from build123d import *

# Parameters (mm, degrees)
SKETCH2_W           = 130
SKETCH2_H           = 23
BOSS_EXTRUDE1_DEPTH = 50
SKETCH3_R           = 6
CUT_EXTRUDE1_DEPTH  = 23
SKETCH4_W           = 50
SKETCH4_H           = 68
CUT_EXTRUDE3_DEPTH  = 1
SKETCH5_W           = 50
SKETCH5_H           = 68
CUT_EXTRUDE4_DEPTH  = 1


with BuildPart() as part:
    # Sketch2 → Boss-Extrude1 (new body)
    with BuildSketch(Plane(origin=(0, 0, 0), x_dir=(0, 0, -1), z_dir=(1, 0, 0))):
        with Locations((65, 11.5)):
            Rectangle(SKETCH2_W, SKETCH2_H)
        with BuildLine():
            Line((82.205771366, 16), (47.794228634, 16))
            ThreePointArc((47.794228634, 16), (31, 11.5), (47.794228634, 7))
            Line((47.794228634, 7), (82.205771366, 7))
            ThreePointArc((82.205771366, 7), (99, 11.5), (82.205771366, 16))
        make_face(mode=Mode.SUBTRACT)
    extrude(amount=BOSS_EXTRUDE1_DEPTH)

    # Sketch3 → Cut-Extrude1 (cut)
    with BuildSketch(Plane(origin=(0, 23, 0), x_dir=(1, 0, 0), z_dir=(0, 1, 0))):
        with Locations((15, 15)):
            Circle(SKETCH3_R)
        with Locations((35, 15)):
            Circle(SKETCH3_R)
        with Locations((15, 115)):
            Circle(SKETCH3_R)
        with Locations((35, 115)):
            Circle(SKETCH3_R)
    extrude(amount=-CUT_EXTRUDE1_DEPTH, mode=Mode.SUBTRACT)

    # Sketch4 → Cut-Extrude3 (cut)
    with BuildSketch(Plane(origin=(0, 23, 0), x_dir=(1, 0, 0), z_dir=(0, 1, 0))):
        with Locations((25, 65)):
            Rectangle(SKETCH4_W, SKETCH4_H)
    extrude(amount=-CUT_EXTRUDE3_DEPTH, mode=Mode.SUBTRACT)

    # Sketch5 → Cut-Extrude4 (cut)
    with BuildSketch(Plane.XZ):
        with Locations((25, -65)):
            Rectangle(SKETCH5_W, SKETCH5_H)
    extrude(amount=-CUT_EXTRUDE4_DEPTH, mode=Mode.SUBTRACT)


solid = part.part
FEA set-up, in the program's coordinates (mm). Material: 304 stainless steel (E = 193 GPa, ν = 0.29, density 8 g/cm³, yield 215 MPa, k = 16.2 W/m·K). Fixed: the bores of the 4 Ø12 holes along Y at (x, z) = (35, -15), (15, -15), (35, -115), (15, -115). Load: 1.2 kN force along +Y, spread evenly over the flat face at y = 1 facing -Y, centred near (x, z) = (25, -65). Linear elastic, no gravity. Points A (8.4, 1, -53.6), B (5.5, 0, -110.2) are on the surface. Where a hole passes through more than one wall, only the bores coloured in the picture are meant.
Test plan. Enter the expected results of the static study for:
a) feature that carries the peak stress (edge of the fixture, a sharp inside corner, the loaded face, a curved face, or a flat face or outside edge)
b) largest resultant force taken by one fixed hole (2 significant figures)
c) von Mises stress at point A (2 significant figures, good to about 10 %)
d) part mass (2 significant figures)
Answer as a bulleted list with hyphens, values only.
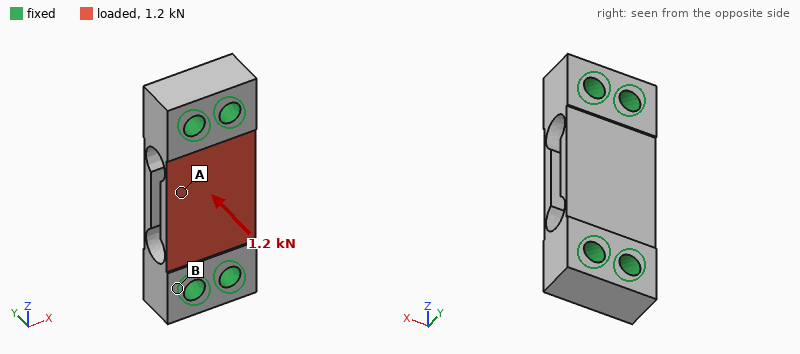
- the loaded face
- 340 N
- 12 MPa
- 740 g
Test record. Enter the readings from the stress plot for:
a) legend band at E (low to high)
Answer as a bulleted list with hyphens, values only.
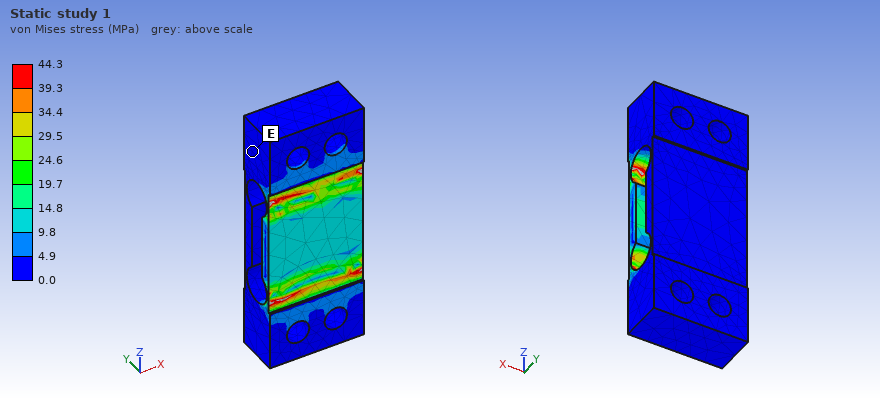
- 0.0 to 4.9 MPa
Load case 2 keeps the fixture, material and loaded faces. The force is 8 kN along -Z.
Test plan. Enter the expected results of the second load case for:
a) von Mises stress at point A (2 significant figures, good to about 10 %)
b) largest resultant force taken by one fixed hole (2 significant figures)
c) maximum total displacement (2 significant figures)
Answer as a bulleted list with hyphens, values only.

- 13 MPa
- 2.0 kN
- 4.9 µm
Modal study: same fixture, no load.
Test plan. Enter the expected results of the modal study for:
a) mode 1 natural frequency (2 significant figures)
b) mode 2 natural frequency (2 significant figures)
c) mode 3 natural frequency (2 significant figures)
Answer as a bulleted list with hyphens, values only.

- 4000 Hz
- 4100 Hz
- 4400 Hz
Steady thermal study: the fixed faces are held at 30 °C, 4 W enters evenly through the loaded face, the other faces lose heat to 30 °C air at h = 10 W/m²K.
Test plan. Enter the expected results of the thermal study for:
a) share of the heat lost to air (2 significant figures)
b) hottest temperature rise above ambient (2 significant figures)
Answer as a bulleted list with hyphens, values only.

- 14 %
- 15 K
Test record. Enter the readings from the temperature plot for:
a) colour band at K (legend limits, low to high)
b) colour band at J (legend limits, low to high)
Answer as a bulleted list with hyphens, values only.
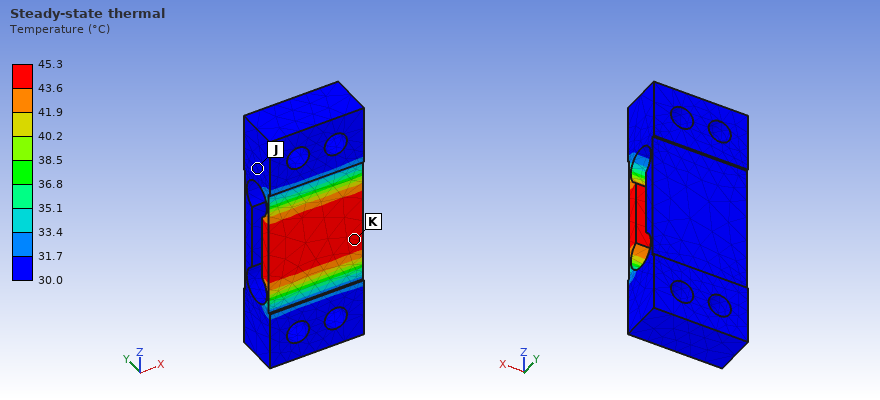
- 43.6 to 45.3 °C
- 30.0 to 31.7 °C
